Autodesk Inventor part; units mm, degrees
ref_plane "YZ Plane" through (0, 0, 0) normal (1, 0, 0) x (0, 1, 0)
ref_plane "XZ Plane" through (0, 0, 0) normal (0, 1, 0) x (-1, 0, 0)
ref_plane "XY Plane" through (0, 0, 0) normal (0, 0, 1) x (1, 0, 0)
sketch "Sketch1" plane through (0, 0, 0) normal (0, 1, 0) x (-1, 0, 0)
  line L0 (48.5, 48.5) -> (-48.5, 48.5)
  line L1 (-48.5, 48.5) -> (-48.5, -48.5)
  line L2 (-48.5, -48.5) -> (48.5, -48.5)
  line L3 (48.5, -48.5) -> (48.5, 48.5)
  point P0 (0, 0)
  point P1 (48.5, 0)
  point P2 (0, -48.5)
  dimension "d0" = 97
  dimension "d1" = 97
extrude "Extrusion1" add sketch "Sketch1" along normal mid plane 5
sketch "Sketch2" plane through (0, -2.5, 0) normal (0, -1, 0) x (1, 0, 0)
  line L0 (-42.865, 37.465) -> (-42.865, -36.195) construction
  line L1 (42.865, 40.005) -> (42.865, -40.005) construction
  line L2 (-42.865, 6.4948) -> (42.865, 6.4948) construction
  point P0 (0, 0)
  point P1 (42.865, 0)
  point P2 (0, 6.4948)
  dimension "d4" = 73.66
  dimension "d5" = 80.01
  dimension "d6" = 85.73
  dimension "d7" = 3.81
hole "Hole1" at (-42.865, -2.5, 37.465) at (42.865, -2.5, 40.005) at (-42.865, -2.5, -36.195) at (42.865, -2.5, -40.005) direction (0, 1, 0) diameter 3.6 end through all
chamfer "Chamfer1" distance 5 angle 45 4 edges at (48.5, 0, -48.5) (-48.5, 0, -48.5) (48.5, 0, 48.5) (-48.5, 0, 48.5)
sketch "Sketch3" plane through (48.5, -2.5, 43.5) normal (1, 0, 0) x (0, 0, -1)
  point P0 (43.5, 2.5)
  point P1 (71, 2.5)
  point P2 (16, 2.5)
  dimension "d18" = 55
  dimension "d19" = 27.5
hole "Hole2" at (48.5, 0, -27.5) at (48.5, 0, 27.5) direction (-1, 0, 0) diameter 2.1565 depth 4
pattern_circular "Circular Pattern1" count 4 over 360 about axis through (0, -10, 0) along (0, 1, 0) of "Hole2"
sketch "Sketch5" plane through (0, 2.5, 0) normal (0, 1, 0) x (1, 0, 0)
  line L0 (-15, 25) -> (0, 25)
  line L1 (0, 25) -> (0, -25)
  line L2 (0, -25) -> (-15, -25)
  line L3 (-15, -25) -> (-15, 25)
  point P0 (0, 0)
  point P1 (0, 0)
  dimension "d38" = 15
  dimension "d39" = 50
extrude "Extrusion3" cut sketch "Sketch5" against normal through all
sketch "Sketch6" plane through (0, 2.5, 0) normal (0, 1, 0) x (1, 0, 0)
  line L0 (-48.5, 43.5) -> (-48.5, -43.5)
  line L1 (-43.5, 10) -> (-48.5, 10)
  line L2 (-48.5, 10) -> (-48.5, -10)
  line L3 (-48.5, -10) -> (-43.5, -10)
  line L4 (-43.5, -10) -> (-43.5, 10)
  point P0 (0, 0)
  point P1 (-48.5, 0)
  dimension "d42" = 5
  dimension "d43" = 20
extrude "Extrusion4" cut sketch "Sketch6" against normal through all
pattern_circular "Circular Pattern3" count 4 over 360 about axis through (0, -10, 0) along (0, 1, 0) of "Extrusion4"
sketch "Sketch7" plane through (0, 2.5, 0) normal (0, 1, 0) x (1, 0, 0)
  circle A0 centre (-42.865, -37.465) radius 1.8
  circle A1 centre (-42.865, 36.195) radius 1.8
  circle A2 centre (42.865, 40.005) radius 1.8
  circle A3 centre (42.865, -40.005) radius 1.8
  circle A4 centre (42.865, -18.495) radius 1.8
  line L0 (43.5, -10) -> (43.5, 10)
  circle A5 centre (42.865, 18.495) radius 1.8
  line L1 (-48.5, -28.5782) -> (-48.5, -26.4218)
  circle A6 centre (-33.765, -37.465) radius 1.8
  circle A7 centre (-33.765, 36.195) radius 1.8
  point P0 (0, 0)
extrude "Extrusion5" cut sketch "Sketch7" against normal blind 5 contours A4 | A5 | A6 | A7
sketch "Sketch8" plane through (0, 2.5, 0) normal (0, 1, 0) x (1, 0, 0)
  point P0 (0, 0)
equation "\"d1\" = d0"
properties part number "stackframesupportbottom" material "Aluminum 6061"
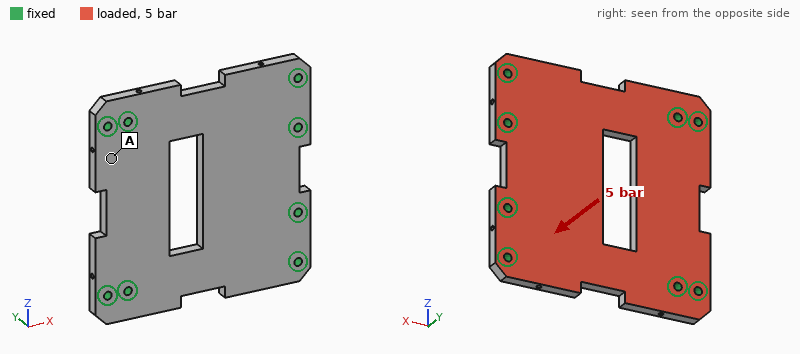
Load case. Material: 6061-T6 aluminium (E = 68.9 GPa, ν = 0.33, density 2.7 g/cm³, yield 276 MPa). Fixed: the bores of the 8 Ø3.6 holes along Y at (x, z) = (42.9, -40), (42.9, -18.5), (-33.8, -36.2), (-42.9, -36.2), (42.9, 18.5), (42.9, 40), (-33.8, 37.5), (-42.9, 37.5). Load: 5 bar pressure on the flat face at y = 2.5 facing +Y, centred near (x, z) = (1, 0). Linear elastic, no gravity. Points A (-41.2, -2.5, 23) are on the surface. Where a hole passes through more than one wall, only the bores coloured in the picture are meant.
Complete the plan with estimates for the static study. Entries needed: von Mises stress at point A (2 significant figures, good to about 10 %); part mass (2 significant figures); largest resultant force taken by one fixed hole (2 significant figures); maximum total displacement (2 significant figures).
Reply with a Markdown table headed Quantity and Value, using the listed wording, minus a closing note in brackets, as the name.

| Quantity | Value |
|---|---|
| von Mises stress at point A | 18 MPa |
| part mass | 110 g |
| largest resultant force taken by one fixed hole | 1.2 kN |
| maximum total displacement | 0.15 mm |
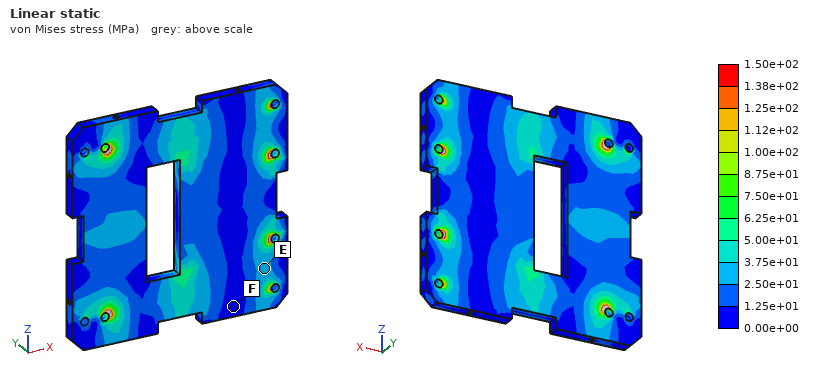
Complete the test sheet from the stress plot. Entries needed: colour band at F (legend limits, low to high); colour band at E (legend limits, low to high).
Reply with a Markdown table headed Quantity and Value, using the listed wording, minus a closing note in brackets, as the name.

| Quantity | Value |
|---|---|
| colour band at F | 0.00e+00 to 1.25e+01 MPa |
| colour band at E | 2.50e+01 to 3.75e+01 MPa |
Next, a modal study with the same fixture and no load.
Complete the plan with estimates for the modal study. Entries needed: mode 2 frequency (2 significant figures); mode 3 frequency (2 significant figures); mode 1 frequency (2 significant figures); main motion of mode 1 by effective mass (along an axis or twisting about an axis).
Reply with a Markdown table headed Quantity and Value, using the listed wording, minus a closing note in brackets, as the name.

| Quantity | Value |
|---|---|
| mode 2 frequency | 4800 Hz |
| mode 3 frequency | 4800 Hz |
| mode 1 frequency | 3400 Hz |
| main motion of mode 1 by effective mass | along Y |
